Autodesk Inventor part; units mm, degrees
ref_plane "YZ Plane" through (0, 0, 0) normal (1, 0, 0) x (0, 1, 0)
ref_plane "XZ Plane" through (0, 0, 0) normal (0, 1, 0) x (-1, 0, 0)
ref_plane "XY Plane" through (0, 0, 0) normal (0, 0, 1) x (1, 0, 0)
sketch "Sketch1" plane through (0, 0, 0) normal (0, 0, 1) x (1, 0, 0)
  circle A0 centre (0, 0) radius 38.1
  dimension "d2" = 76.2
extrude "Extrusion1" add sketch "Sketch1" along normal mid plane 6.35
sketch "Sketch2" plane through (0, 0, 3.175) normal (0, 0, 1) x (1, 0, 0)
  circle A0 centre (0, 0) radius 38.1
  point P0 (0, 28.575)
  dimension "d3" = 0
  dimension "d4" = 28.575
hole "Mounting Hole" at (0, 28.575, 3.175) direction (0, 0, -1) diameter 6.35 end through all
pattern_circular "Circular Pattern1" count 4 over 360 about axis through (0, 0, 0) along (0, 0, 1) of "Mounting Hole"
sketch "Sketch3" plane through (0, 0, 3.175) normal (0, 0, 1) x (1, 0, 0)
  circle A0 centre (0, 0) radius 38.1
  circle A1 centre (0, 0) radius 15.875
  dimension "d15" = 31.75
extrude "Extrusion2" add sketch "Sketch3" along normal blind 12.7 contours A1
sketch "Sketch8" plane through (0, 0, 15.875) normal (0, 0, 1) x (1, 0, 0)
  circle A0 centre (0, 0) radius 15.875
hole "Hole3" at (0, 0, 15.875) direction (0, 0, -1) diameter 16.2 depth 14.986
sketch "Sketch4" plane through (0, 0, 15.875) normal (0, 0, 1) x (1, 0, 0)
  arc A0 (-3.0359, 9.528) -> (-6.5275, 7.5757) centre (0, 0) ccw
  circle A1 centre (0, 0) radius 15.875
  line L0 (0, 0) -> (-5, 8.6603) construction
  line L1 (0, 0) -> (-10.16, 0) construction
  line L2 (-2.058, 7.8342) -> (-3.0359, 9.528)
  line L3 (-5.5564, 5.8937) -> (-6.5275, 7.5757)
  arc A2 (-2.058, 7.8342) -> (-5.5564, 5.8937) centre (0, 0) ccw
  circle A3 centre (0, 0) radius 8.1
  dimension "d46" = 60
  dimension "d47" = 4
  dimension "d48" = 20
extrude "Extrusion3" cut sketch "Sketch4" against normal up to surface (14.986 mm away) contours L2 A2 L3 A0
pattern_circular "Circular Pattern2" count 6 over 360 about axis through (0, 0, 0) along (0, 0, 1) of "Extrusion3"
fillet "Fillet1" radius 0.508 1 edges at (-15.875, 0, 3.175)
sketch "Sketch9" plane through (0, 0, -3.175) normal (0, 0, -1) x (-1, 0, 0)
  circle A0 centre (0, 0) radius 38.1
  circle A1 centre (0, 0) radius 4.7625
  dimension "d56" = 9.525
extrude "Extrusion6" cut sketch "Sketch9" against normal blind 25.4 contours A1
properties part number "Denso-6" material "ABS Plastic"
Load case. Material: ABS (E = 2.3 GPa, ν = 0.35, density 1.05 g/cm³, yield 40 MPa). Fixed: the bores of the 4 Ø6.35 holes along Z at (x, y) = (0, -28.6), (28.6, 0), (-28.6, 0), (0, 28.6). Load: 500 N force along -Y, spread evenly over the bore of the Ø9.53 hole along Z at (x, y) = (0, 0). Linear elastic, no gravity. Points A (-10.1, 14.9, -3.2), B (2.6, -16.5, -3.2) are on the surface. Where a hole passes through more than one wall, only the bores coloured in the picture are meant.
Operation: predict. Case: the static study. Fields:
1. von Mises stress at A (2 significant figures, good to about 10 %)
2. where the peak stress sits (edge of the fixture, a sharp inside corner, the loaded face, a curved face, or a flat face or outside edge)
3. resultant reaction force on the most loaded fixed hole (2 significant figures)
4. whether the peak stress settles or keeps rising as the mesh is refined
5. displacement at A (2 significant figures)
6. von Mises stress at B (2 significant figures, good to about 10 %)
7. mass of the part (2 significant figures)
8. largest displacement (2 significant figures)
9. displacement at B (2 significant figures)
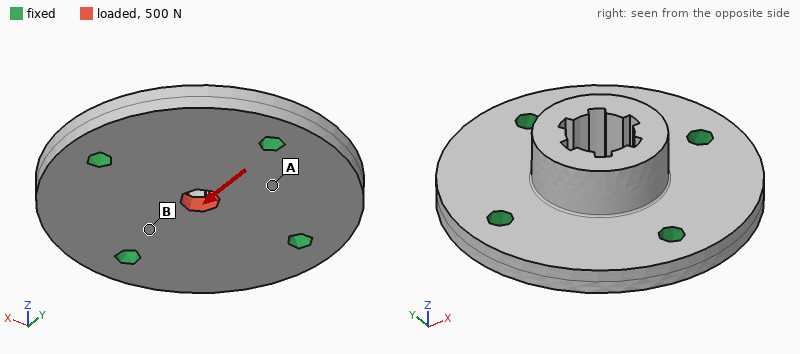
1.1 MPa
a sharp inside corner
170 N
keeps rising
8.8 µm
2.2 MPa
36 g
26 µm
8.4 µm
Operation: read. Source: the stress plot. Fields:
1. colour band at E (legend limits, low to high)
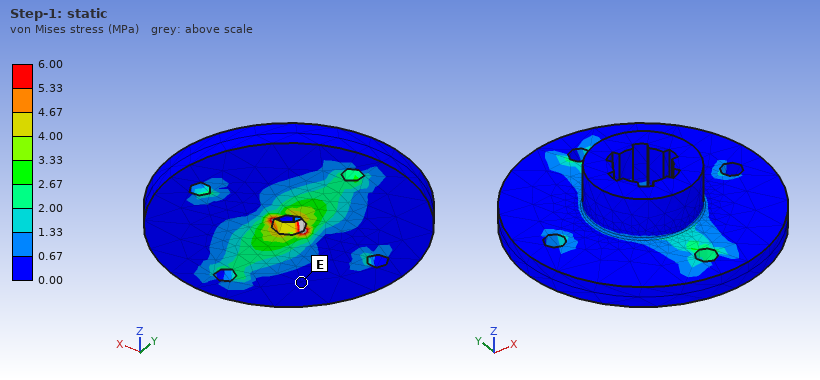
0.00 to 0.67 MPa
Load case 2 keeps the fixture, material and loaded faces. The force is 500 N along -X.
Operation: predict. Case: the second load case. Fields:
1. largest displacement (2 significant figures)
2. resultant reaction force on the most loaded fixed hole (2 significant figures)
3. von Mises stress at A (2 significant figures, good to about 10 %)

26 µm
170 N
0.67 MPa
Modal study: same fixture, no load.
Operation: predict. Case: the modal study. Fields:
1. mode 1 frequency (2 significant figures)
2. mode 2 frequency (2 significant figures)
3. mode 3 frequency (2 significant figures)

4100 Hz
4100 Hz
4100 Hz
